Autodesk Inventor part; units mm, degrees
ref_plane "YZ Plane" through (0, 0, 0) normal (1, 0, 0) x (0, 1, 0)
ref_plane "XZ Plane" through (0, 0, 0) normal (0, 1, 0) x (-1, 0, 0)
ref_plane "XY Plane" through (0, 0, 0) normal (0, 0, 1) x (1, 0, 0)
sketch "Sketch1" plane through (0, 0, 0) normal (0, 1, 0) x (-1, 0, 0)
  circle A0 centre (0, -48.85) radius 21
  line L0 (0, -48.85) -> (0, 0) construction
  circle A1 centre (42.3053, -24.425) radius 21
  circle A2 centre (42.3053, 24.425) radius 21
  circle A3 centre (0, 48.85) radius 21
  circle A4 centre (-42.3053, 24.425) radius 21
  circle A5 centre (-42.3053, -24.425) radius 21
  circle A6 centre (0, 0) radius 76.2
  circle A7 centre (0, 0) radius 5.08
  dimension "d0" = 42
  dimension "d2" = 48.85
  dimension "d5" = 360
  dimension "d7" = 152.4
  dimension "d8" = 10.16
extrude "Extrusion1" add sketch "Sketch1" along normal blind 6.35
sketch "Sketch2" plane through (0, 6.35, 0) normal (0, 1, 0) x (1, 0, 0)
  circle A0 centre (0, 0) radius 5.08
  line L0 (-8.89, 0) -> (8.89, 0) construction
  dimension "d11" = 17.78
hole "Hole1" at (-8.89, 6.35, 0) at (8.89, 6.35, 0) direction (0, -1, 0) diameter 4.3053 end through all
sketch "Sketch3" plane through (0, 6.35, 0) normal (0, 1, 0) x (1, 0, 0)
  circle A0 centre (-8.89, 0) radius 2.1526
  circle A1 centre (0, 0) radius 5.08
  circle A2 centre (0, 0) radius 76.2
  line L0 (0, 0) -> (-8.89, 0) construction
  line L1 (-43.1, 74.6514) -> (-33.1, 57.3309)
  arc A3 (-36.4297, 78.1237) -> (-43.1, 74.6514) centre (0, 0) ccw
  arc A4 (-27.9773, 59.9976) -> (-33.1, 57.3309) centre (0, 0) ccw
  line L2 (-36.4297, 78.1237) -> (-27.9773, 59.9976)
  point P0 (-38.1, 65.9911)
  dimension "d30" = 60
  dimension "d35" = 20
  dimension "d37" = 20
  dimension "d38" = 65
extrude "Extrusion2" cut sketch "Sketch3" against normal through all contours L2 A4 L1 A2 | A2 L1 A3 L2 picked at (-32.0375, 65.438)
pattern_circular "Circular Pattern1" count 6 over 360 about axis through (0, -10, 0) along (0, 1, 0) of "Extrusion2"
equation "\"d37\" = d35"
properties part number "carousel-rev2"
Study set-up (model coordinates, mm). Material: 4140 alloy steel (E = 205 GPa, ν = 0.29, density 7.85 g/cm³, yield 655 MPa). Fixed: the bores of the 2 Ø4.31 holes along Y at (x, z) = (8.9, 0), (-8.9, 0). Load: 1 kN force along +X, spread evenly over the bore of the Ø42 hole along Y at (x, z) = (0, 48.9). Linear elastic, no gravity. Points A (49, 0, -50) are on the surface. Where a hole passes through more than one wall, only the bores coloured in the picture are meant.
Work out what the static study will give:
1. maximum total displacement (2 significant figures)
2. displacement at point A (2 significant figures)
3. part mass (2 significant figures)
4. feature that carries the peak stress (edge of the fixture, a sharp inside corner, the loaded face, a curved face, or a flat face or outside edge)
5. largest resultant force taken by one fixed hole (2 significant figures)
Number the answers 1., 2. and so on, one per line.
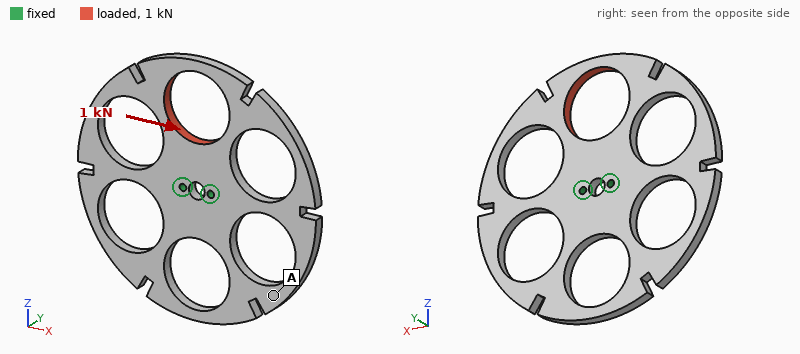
1. 27 µm
2. 16 µm
3. 470 g
4. edge of the fixture
5. 2.3 kN
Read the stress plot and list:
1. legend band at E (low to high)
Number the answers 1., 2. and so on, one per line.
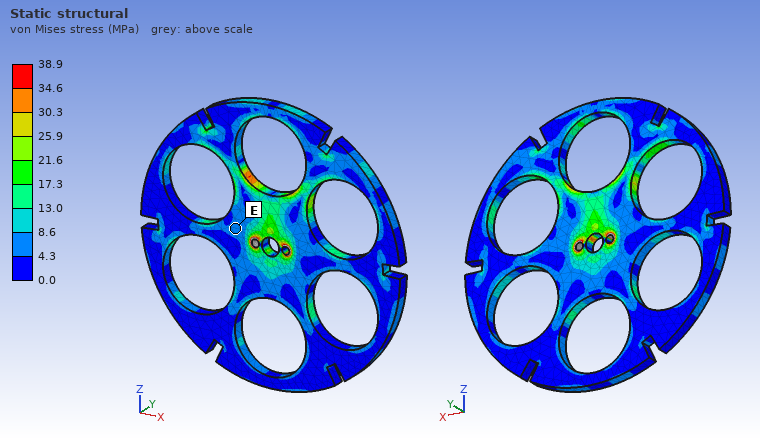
1. 4.3 to 8.6 MPa
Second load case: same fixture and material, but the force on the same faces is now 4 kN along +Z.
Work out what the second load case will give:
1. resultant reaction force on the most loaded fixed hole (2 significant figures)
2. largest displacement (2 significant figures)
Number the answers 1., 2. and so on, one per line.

1. 2.0 kN
2. 24 µm
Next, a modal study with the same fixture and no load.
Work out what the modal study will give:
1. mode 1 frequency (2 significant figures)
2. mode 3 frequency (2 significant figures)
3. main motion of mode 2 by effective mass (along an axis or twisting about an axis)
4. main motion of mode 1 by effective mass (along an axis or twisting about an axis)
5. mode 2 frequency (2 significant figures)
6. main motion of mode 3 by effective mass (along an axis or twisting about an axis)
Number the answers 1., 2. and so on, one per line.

1. 710 Hz
2. 870 Hz
3. twisting about Z
4. twisting about X
5. 830 Hz
6. along Y
